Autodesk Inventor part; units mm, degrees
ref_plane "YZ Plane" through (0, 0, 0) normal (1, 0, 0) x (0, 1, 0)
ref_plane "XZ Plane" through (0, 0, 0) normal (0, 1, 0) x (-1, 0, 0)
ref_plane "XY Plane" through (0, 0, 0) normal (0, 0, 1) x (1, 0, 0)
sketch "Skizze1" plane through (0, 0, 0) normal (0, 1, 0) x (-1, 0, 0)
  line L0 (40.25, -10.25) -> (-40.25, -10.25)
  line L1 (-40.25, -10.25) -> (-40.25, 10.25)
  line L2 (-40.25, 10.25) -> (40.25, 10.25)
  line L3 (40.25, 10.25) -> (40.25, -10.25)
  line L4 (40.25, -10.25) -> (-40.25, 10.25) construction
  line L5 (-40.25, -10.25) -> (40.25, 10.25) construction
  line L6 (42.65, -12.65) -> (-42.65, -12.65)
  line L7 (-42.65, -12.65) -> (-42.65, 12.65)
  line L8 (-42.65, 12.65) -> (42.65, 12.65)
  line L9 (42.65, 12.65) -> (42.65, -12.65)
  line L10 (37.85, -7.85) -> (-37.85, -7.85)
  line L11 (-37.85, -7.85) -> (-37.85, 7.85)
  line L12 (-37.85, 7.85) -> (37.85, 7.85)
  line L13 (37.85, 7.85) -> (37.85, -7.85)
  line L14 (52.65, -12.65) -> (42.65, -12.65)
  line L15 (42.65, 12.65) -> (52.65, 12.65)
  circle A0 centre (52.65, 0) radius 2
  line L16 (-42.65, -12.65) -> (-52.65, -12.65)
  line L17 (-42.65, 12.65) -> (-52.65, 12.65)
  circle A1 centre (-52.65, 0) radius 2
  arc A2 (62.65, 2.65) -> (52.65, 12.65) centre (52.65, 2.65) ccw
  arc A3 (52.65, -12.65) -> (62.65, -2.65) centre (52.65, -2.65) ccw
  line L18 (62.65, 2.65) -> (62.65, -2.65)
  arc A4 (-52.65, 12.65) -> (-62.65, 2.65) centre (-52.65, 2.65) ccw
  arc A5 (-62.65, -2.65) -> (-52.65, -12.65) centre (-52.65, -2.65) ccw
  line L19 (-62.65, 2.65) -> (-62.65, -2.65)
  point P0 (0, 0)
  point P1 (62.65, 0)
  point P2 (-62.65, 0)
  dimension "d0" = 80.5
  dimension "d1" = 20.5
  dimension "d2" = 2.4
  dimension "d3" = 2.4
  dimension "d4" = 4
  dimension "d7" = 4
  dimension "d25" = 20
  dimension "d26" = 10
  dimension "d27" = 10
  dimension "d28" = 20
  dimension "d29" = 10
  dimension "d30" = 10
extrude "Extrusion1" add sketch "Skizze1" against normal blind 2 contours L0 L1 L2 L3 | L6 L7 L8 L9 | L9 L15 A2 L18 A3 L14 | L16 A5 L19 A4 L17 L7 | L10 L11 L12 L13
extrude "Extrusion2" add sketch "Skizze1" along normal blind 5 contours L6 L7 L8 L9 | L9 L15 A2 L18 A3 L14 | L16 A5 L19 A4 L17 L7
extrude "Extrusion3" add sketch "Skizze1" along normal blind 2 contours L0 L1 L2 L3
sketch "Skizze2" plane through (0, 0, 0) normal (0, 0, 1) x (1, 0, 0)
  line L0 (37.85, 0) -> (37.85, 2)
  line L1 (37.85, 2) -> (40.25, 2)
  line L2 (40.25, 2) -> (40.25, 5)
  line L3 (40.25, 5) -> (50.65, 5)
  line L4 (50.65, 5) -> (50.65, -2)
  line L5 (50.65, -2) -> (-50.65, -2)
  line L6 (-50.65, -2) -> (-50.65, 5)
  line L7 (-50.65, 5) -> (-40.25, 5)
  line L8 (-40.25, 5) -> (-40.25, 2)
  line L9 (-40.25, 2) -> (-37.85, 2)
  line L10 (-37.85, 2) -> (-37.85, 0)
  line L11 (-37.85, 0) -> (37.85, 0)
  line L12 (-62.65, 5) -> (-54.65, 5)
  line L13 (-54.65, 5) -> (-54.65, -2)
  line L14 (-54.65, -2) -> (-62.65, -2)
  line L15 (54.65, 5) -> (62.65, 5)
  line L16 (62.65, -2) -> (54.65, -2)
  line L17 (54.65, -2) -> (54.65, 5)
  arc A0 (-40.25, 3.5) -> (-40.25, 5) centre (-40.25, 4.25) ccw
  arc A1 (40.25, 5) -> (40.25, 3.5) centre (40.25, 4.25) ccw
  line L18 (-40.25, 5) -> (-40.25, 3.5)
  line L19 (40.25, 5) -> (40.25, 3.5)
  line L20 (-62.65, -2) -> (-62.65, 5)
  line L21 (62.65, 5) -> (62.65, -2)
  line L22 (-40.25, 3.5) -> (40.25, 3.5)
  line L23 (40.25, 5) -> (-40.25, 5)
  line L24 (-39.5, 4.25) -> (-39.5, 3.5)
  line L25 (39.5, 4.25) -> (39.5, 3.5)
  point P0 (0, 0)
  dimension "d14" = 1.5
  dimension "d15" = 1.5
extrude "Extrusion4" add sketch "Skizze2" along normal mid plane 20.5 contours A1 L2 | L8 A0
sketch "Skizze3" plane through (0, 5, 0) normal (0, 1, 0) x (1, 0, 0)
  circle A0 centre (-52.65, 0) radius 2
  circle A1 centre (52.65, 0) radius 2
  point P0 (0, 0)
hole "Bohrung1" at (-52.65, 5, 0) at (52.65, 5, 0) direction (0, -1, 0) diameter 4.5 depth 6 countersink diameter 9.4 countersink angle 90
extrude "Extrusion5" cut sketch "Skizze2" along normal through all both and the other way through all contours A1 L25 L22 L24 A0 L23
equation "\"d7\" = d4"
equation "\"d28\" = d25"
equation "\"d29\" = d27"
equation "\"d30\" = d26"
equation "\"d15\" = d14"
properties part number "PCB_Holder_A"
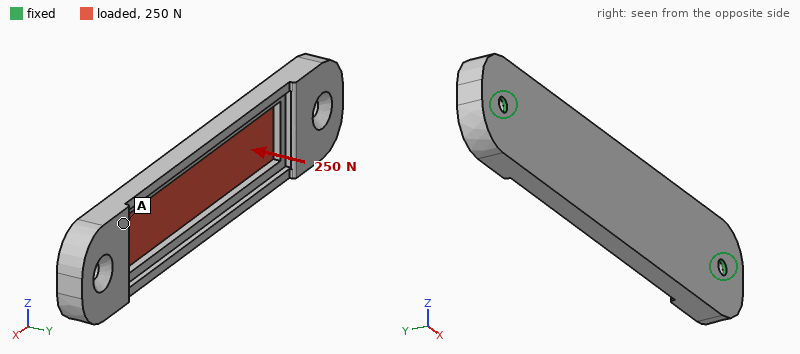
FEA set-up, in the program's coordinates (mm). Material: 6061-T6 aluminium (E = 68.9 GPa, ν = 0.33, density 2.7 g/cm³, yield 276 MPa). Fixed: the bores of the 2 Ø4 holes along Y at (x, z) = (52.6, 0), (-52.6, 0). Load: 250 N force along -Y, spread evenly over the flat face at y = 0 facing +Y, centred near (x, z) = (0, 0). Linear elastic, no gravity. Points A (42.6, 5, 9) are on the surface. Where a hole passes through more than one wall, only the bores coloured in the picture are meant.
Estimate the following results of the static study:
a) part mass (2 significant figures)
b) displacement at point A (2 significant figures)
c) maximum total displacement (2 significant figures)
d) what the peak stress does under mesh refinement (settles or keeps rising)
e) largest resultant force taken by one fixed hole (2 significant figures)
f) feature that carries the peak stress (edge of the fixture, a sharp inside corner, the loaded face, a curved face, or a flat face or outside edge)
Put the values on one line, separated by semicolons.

36 g; 0.033 mm; 0.14 mm; keeps rising; 320 N; edge of the fixture
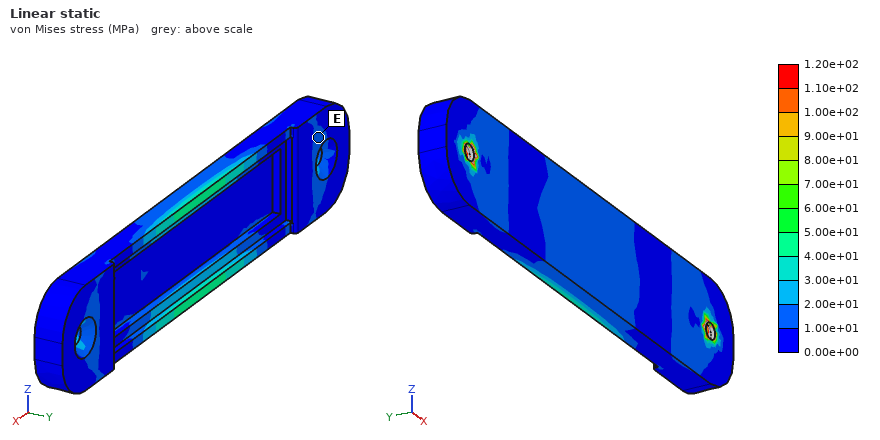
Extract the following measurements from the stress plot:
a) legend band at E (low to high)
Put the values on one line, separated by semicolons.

1.00e+01 to 2.00e+01 MPa
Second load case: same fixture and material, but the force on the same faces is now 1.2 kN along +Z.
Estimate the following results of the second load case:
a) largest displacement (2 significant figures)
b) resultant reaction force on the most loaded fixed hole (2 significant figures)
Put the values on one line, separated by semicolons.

92 µm; 600 N
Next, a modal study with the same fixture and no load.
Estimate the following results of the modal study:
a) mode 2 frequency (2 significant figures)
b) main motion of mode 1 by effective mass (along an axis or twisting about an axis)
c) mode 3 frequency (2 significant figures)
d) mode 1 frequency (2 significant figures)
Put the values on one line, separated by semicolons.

3200 Hz; along Y; 4500 Hz; 1800 Hz
